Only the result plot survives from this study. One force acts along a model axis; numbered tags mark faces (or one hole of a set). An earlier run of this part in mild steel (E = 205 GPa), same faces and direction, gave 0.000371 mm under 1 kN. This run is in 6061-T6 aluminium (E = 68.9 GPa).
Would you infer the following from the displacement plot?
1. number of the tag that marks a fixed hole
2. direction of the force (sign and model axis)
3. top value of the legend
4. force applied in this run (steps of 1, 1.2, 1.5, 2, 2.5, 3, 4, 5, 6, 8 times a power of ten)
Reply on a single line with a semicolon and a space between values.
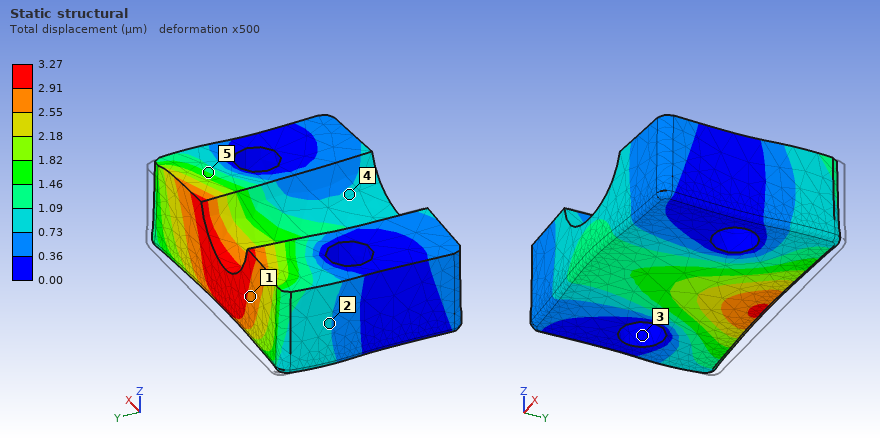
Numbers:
3; -Y; 3.27 µm; 3 kN
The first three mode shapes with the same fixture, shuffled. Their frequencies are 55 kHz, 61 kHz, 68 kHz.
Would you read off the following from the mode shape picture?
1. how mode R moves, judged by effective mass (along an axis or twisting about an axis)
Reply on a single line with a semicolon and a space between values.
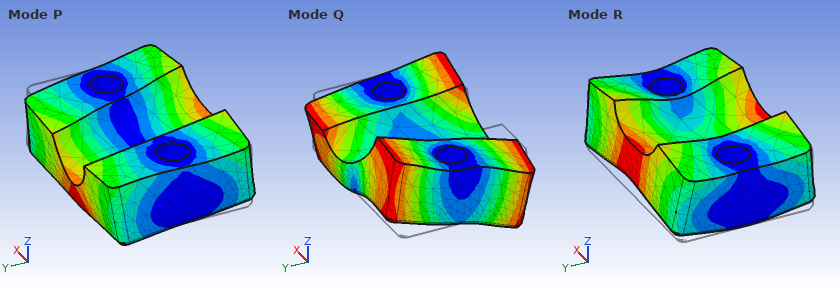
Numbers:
along Z
